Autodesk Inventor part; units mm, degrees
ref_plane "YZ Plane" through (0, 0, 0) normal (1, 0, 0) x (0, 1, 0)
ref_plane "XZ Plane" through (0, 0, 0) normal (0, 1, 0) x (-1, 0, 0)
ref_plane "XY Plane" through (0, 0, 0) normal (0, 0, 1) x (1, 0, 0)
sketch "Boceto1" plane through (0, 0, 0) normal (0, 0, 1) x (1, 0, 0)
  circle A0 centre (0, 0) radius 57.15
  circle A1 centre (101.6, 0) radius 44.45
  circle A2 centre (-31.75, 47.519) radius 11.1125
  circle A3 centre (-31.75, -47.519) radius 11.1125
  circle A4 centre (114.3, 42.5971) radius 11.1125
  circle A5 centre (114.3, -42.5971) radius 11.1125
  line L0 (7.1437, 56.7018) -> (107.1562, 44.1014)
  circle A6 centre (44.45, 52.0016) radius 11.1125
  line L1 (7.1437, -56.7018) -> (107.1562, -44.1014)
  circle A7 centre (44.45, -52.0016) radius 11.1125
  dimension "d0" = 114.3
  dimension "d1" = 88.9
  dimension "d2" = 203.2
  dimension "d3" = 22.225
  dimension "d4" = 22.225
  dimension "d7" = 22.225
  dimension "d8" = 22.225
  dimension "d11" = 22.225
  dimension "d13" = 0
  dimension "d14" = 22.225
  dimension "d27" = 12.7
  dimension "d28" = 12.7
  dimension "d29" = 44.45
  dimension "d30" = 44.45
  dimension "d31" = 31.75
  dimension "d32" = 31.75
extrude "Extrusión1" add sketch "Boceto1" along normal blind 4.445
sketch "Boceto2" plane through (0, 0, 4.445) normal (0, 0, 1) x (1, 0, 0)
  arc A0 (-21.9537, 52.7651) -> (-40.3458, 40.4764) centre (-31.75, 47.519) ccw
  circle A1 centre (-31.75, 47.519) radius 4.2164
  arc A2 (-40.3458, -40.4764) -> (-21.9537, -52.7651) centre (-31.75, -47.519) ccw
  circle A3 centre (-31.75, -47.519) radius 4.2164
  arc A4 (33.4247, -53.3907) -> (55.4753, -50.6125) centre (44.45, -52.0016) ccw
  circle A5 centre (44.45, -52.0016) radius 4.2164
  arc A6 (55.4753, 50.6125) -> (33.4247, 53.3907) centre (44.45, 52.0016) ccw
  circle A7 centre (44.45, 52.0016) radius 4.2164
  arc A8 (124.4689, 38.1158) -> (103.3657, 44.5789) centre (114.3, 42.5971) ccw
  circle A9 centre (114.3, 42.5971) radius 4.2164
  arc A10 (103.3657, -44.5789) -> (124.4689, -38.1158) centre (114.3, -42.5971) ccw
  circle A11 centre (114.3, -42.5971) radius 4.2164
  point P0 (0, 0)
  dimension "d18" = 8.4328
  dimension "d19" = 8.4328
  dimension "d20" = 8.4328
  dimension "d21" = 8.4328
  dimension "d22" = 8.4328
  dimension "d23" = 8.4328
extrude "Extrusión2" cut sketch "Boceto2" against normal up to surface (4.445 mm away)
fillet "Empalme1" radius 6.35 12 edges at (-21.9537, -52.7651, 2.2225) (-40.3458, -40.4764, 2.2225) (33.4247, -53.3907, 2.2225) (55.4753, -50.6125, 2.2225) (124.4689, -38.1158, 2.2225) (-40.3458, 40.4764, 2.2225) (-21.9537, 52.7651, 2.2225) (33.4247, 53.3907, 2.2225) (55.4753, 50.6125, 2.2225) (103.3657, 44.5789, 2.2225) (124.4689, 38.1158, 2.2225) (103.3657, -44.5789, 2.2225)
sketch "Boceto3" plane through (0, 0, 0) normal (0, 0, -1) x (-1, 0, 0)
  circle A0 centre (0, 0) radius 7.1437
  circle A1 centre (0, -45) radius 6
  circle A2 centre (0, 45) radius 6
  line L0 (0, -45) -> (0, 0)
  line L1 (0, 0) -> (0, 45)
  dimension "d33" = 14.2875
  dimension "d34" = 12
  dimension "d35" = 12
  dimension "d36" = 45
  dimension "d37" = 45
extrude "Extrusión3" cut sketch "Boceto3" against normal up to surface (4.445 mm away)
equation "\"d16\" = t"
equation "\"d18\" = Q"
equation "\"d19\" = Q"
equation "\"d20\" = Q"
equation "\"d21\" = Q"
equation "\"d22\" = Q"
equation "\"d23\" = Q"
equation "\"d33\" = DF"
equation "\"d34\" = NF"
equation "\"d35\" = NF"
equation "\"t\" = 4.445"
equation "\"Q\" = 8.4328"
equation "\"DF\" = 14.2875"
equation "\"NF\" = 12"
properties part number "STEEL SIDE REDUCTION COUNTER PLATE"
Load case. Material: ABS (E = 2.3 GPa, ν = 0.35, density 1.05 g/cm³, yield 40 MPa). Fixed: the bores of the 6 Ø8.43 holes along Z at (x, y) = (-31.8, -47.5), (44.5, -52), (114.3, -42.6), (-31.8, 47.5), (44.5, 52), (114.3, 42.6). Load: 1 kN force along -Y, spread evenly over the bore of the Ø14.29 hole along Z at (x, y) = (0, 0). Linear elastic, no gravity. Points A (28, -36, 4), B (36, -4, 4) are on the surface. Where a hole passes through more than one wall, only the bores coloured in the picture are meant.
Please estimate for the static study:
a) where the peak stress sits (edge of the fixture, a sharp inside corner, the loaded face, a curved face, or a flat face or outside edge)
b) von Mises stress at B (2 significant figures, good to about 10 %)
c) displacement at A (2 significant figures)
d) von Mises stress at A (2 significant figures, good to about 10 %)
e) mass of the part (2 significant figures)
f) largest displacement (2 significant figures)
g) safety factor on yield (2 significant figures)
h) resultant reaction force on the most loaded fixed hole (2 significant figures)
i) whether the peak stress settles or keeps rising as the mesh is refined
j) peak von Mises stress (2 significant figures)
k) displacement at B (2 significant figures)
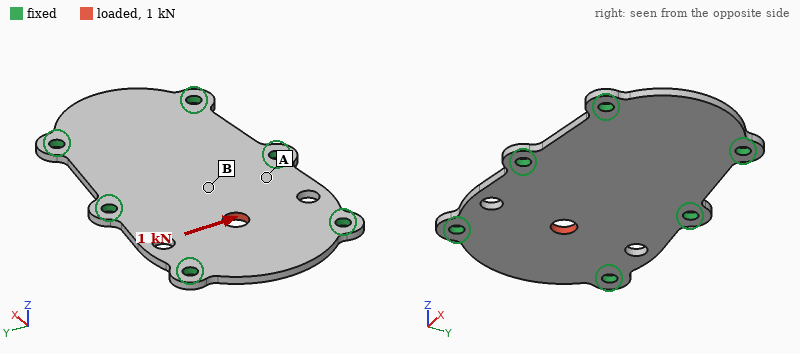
the loaded face
0.87 MPa
25 µm
2.1 MPa
89 g
77 µm
4.6
300 N
settles
8.7 MPa
23 µm
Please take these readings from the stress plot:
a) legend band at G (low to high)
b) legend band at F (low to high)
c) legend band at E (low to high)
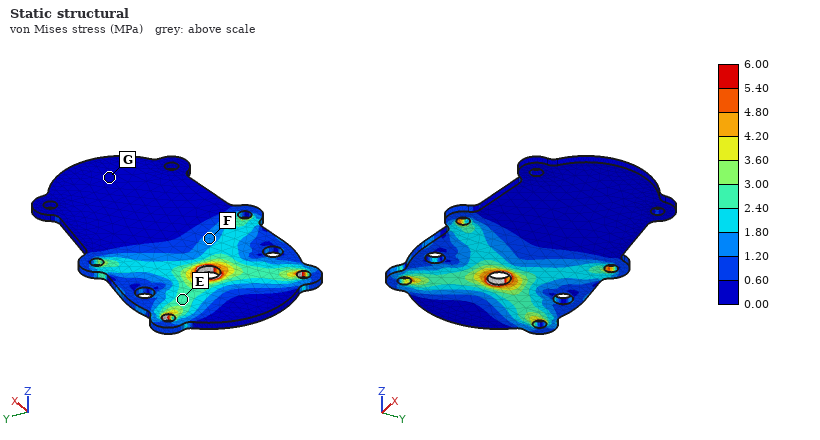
0.00 to 0.60 MPa
1.20 to 1.80 MPa
2.40 to 3.00 MPa
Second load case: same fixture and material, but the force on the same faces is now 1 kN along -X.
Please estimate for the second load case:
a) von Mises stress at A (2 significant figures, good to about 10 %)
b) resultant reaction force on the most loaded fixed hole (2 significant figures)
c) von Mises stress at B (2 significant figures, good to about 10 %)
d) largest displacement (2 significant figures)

1.8 MPa
230 N
1.7 MPa
88 µm
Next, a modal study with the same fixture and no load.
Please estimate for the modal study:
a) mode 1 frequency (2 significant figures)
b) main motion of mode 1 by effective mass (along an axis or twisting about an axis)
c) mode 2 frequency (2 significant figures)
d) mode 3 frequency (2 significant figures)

600 Hz
along Z
720 Hz
740 Hz
